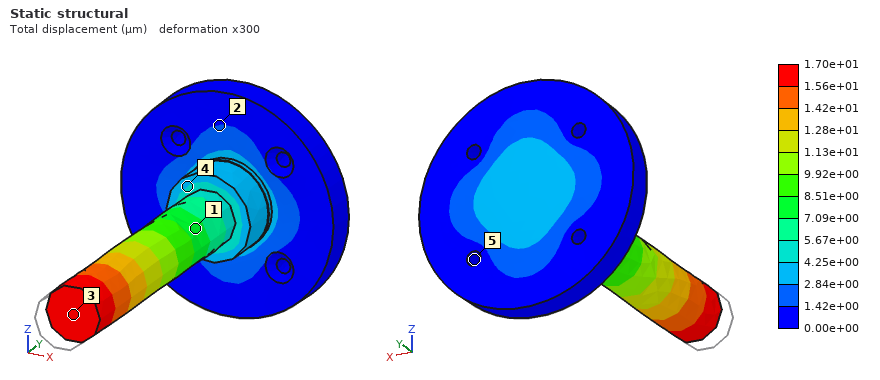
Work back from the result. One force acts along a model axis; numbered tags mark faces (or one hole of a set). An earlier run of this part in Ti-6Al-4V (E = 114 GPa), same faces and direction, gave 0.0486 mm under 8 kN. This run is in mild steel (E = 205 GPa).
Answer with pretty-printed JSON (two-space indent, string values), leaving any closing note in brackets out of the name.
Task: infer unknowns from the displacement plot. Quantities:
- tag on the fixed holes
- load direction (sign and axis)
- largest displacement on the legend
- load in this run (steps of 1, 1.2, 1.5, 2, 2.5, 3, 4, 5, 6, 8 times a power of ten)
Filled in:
{
  "tag on the fixed holes": "5",
  "load direction": "+Y",
  "largest displacement on the legend": "1.70e+01 µm",
  "load in this run": "5 kN"
}
